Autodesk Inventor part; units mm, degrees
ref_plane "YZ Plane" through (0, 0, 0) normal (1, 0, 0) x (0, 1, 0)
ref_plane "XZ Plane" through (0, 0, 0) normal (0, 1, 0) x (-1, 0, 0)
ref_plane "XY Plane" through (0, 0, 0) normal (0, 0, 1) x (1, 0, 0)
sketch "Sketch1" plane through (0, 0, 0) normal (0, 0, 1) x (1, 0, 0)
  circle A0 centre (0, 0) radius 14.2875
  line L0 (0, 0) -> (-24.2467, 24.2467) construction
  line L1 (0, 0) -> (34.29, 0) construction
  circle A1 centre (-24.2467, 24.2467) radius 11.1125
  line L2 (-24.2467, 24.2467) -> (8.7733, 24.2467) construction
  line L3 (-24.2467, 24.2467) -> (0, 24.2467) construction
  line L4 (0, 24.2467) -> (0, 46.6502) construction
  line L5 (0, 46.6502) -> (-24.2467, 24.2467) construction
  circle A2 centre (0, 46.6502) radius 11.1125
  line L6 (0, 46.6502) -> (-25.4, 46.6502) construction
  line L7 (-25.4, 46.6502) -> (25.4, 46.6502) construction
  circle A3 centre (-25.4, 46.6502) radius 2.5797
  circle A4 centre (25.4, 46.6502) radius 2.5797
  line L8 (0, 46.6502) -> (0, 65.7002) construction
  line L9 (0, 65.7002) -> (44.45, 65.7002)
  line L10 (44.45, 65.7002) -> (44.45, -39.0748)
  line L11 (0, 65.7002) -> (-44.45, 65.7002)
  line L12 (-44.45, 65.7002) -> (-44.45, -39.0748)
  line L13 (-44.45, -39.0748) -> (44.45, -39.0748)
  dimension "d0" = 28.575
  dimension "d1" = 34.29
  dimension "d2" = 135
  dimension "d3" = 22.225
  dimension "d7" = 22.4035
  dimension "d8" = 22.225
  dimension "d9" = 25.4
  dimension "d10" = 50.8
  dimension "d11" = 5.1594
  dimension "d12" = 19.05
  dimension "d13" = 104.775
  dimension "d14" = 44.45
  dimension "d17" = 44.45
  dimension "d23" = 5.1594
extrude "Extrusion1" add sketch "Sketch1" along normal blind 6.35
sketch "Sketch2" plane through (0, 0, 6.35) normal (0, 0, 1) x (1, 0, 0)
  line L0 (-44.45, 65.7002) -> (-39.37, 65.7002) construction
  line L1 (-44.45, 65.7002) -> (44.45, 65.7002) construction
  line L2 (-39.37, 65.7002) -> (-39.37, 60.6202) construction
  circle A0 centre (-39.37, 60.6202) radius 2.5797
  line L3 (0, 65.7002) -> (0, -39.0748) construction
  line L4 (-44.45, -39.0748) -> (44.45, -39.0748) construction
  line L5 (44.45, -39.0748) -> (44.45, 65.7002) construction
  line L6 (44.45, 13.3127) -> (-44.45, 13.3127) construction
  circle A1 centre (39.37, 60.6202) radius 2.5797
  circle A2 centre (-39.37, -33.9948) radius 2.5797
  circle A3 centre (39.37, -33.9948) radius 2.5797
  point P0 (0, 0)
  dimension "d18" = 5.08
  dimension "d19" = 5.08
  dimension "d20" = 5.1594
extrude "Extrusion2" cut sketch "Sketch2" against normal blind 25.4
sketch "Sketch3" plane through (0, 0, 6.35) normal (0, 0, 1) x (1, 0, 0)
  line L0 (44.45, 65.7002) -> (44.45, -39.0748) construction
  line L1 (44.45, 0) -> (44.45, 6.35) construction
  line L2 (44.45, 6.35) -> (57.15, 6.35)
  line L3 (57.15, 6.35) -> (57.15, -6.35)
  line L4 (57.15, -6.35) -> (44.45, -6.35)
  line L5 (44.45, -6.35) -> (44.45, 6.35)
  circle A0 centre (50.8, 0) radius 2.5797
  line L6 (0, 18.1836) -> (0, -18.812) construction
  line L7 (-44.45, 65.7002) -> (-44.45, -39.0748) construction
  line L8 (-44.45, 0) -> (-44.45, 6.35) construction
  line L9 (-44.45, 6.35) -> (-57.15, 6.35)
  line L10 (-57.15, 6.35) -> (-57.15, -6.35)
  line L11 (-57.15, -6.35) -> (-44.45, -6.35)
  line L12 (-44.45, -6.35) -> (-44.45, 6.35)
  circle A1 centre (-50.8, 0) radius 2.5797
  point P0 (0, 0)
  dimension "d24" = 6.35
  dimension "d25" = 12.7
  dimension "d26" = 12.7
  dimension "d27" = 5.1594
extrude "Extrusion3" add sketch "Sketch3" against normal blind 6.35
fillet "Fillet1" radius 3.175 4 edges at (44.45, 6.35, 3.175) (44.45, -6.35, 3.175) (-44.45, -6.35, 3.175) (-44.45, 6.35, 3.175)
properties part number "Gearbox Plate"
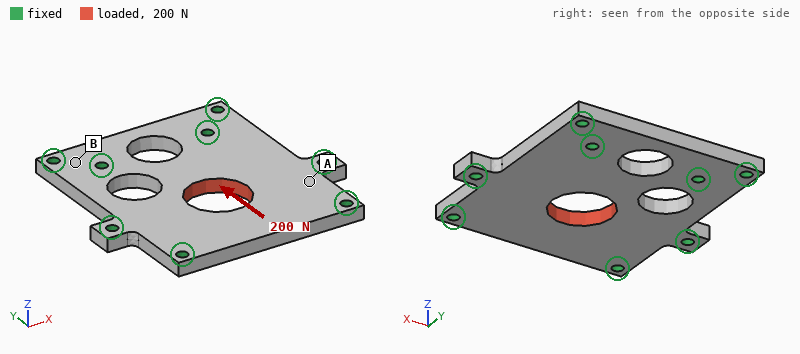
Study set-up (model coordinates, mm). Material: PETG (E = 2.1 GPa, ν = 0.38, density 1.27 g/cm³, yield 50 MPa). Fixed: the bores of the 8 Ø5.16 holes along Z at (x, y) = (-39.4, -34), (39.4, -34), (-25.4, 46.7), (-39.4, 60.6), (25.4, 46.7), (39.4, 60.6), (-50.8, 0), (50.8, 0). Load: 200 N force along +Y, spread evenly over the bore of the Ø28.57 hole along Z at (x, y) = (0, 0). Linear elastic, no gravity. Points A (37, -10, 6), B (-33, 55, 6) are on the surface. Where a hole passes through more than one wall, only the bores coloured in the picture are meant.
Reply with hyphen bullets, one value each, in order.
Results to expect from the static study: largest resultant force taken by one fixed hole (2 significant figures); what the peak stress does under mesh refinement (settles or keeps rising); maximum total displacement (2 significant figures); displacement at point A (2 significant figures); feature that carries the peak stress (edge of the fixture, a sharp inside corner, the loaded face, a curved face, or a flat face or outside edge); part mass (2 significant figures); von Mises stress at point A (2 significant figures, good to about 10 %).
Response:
- 54 N
- keeps rising
- 14 µm
- 2.5 µm
- edge of the fixture
- 65 g
- 0.25 MPa
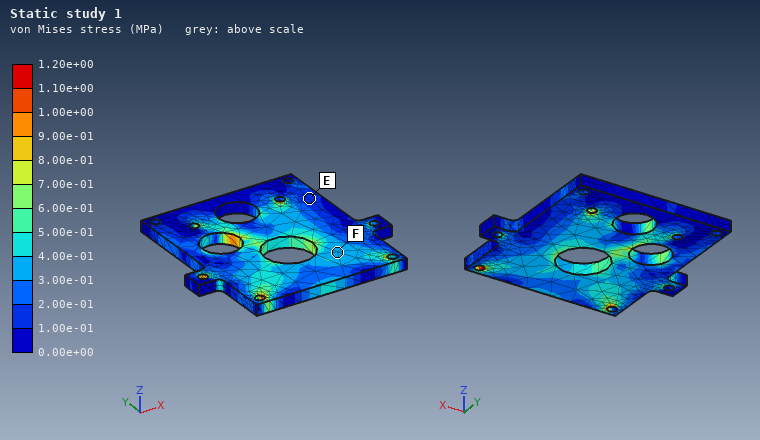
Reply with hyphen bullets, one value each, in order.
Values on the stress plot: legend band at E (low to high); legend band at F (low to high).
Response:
- 1.00e-01 to 2.00e-01 MPa
- 3.00e-01 to 4.00e-01 MPa
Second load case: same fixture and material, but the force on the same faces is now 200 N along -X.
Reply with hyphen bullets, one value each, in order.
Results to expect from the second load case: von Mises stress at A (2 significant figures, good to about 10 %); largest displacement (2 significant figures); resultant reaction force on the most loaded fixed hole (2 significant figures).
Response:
- 0.18 MPa
- 9.6 µm
- 51 N
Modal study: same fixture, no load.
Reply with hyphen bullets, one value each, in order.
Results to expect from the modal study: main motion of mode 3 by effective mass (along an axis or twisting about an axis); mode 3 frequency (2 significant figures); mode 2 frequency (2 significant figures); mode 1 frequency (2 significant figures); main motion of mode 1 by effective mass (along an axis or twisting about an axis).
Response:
- twisting about Y
- 2200 Hz
- 1700 Hz
- 1100 Hz
- along Z
